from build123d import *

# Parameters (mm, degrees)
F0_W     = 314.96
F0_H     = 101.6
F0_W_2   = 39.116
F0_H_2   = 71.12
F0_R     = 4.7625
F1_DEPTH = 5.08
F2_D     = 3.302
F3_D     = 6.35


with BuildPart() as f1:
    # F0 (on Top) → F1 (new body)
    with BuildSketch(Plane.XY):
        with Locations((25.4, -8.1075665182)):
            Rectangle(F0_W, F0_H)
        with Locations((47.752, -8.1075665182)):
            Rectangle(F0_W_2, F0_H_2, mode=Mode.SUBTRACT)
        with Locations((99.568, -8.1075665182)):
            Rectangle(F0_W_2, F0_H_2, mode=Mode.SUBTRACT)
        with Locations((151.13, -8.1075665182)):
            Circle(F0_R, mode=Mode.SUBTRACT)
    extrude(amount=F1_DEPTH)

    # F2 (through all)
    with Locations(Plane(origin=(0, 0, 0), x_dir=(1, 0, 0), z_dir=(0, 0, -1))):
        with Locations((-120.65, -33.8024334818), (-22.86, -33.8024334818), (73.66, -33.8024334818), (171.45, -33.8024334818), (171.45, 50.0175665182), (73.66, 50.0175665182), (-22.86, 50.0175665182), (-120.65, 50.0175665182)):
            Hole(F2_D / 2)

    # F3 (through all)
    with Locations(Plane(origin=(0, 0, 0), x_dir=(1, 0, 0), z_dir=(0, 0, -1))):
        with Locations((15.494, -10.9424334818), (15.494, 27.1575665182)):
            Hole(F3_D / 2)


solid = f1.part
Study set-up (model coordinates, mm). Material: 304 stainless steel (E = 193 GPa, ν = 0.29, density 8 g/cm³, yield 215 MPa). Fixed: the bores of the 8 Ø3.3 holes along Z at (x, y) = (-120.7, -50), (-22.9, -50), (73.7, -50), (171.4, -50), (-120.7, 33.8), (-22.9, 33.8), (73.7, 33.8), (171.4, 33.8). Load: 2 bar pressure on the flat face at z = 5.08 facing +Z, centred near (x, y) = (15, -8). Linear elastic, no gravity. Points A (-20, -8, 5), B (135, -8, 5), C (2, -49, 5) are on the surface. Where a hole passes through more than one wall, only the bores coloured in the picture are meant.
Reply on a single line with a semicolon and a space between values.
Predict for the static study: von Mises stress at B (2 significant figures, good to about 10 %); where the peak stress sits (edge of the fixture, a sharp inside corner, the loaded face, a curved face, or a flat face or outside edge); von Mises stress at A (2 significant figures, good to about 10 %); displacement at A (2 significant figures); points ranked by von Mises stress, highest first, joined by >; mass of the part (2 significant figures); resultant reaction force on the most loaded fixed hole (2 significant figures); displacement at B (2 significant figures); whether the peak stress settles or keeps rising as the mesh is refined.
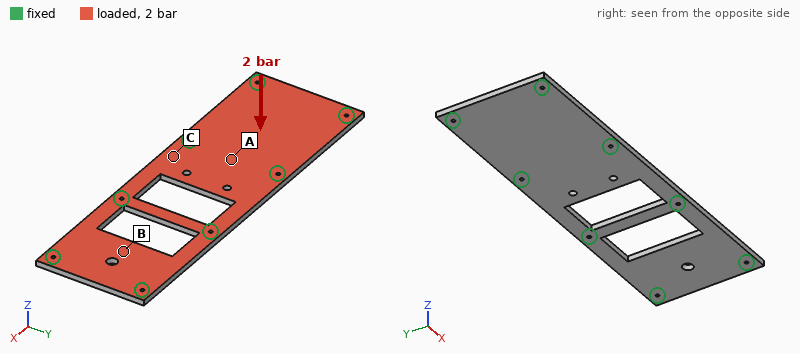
20 MPa; edge of the fixture; 29 MPa; 31 µm; A > B > C; 1.1 kg; 980 N; 58 µm; keeps rising
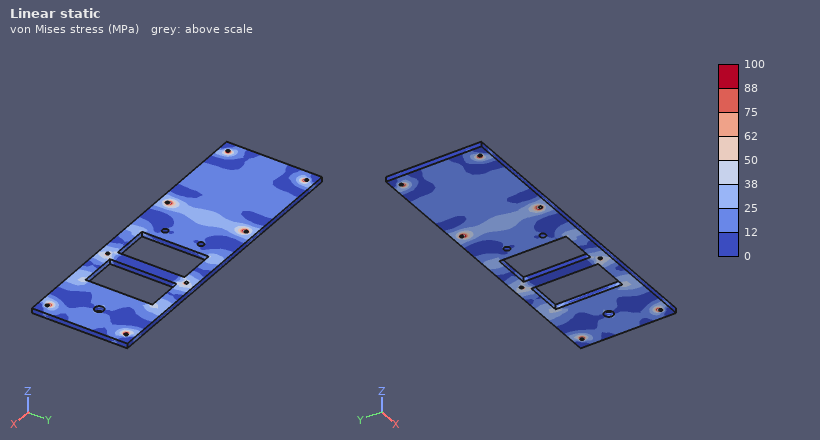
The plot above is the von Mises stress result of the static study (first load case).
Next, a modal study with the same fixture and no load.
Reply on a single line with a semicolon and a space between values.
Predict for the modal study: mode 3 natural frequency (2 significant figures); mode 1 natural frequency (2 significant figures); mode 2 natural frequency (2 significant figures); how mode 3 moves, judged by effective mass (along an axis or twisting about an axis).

1900 Hz; 1700 Hz; 1800 Hz; along Z
